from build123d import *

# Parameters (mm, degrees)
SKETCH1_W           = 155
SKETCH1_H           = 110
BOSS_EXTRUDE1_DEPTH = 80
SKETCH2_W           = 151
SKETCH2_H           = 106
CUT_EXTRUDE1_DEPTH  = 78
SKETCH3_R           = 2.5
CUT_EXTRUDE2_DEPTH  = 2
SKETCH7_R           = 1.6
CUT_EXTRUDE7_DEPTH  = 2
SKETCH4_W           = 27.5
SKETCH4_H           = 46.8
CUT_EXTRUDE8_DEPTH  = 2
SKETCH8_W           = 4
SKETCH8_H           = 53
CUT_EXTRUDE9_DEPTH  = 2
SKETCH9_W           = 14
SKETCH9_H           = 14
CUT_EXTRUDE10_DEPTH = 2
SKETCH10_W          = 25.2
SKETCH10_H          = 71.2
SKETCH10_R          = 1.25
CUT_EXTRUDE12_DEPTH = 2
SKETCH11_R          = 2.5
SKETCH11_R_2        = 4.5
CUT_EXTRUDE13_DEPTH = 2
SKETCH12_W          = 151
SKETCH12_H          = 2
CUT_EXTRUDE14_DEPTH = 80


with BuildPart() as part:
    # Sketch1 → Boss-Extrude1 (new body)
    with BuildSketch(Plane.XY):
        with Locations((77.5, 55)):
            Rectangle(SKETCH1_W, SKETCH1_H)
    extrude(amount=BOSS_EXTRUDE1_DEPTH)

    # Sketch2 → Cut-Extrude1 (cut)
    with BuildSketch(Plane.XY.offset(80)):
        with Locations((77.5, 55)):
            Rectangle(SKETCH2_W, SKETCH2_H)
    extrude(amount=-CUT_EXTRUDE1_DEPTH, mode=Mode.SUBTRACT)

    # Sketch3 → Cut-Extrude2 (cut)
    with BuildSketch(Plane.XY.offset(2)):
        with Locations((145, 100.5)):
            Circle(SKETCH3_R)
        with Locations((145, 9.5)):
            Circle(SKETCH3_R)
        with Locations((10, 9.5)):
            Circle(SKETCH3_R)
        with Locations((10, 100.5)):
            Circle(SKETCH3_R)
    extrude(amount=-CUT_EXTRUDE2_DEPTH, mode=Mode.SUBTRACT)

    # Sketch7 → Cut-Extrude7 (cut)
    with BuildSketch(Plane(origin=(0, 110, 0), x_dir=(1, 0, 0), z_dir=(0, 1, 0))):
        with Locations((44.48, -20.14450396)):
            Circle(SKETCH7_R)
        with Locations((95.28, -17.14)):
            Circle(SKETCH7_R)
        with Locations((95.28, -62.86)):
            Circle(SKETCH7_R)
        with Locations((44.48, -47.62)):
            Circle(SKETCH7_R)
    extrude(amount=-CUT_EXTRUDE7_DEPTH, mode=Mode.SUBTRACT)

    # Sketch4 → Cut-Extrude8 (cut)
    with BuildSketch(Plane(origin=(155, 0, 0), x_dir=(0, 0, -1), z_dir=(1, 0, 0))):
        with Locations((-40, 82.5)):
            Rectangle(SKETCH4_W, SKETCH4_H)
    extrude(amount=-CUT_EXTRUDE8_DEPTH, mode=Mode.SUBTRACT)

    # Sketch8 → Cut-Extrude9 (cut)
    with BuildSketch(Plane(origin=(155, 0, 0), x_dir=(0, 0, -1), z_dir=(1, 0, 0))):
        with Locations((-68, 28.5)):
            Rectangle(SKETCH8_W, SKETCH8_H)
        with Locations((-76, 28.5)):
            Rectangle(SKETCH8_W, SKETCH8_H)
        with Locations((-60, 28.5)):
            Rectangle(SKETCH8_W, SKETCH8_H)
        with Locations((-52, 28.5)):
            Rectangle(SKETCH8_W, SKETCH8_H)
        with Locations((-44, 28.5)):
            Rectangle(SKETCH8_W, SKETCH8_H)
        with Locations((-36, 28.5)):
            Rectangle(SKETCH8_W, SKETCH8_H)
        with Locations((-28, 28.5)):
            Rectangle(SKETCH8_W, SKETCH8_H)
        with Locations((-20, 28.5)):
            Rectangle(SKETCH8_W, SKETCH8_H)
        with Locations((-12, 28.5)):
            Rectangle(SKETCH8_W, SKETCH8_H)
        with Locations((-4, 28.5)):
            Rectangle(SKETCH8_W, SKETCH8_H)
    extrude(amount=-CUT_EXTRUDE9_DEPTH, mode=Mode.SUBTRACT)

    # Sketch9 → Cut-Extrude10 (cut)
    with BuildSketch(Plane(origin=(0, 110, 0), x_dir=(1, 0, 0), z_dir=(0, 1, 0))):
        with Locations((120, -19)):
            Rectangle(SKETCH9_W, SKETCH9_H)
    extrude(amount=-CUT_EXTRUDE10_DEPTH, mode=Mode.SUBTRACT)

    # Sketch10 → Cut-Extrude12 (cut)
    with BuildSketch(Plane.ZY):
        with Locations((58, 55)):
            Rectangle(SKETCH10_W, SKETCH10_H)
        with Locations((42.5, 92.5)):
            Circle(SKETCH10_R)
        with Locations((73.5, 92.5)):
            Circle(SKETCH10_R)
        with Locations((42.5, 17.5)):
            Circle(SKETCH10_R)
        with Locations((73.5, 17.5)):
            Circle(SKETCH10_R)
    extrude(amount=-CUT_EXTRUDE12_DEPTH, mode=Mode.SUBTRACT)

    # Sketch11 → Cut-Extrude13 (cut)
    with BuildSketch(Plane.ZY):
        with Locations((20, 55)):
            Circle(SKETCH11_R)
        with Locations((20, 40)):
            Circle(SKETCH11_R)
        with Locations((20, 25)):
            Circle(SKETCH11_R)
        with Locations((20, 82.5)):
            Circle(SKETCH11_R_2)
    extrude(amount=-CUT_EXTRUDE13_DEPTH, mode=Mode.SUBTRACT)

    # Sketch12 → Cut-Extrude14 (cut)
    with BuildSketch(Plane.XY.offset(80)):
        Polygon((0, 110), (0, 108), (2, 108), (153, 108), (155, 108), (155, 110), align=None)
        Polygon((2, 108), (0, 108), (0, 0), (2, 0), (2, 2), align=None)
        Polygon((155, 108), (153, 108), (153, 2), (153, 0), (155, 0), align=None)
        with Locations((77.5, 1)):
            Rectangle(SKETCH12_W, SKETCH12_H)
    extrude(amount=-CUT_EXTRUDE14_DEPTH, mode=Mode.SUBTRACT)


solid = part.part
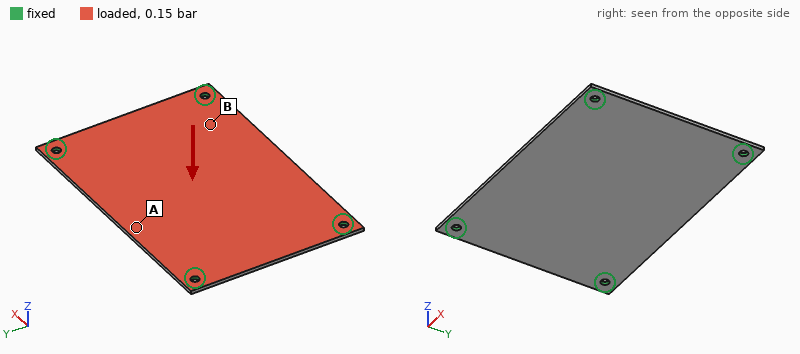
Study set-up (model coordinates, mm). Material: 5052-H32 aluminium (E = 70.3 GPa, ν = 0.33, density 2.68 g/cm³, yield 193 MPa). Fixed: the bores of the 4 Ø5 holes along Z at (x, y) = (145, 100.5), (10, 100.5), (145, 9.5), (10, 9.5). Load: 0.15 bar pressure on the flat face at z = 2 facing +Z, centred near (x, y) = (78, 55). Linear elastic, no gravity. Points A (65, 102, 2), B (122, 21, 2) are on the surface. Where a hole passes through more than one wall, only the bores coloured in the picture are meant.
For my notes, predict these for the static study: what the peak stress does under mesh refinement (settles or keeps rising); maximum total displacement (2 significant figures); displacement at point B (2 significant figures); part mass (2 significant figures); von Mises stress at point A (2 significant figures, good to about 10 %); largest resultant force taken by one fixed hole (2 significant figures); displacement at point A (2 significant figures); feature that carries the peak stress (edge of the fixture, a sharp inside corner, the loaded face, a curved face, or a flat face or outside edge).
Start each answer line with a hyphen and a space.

- keeps rising
- 0.42 mm
- 0.16 mm
- 85 g
- 20 MPa
- 60 N
- 0.35 mm
- edge of the fixture
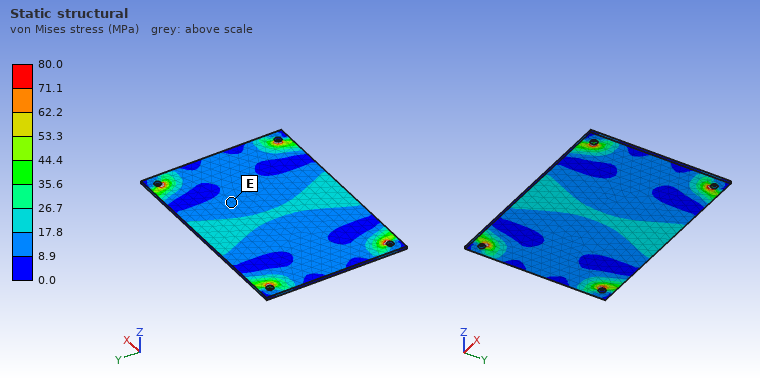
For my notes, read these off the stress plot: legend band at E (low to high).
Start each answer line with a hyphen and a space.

- 8.9 to 17.8 MPa
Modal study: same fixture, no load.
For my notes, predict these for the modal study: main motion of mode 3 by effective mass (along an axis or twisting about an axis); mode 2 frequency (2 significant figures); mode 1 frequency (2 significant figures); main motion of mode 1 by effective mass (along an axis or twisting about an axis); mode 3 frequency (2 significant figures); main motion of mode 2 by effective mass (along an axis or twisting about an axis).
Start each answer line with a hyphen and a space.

- twisting about Y
- 760 Hz
- 480 Hz
- along Z
- 1200 Hz
- twisting about X
